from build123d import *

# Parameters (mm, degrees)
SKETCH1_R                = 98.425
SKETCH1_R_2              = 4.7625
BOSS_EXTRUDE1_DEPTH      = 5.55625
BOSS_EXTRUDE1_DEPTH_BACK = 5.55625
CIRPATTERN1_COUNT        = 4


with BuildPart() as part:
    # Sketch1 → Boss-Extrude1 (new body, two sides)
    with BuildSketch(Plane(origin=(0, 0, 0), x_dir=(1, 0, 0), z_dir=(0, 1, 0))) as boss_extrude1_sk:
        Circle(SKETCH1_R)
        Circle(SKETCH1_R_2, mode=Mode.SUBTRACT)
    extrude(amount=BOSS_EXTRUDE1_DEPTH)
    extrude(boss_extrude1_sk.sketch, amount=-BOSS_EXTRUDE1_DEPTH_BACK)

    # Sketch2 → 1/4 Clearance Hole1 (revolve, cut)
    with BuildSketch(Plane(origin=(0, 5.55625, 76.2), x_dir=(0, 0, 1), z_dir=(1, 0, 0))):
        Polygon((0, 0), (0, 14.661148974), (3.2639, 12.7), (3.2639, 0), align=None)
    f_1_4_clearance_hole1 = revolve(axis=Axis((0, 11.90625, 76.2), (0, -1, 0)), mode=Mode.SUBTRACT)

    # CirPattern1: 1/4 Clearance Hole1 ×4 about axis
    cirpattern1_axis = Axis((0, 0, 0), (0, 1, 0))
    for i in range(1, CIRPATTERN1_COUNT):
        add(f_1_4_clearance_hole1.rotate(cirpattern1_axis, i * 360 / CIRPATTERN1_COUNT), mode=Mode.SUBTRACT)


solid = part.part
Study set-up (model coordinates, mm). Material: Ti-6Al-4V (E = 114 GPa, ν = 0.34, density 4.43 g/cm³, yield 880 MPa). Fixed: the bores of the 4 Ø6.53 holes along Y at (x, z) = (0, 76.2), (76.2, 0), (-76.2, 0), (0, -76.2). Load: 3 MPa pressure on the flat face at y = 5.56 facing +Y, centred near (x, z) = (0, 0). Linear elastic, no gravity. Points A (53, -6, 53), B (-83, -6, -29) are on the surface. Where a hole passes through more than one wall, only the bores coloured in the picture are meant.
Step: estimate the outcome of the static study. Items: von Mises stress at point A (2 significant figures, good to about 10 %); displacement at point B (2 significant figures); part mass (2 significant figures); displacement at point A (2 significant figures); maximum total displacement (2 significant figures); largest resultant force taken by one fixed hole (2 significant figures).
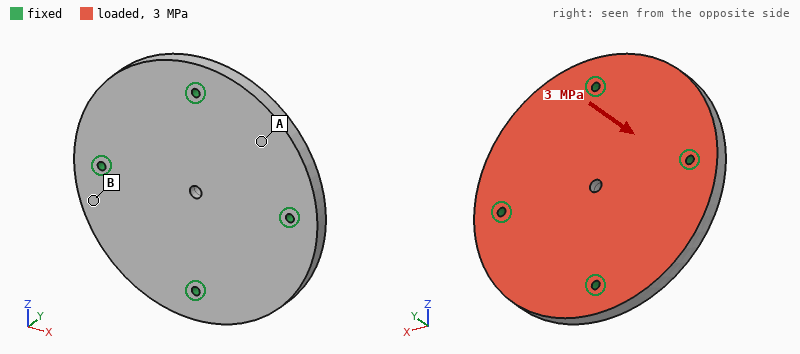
90 MPa
0.071 mm
1.5 kg
0.15 mm
0.21 mm
23 kN
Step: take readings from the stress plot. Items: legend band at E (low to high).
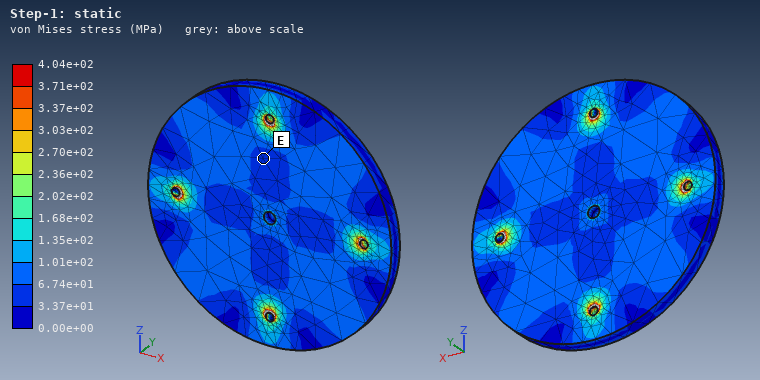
3.37e+01 to 6.74e+01 MPa
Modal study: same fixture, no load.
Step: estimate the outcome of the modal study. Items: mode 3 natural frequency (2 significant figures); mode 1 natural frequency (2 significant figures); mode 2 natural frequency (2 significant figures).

3200 Hz
2800 Hz
3200 Hz
